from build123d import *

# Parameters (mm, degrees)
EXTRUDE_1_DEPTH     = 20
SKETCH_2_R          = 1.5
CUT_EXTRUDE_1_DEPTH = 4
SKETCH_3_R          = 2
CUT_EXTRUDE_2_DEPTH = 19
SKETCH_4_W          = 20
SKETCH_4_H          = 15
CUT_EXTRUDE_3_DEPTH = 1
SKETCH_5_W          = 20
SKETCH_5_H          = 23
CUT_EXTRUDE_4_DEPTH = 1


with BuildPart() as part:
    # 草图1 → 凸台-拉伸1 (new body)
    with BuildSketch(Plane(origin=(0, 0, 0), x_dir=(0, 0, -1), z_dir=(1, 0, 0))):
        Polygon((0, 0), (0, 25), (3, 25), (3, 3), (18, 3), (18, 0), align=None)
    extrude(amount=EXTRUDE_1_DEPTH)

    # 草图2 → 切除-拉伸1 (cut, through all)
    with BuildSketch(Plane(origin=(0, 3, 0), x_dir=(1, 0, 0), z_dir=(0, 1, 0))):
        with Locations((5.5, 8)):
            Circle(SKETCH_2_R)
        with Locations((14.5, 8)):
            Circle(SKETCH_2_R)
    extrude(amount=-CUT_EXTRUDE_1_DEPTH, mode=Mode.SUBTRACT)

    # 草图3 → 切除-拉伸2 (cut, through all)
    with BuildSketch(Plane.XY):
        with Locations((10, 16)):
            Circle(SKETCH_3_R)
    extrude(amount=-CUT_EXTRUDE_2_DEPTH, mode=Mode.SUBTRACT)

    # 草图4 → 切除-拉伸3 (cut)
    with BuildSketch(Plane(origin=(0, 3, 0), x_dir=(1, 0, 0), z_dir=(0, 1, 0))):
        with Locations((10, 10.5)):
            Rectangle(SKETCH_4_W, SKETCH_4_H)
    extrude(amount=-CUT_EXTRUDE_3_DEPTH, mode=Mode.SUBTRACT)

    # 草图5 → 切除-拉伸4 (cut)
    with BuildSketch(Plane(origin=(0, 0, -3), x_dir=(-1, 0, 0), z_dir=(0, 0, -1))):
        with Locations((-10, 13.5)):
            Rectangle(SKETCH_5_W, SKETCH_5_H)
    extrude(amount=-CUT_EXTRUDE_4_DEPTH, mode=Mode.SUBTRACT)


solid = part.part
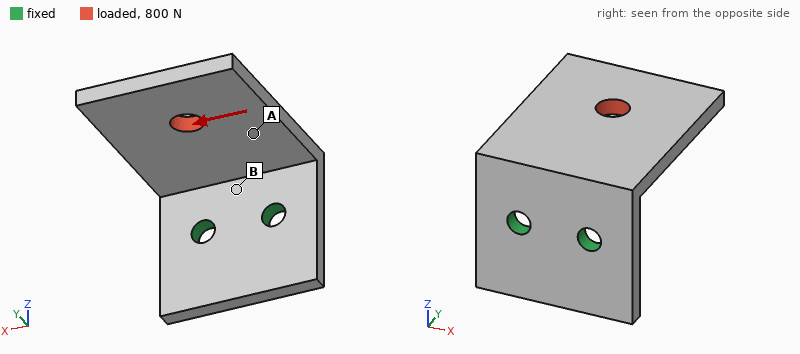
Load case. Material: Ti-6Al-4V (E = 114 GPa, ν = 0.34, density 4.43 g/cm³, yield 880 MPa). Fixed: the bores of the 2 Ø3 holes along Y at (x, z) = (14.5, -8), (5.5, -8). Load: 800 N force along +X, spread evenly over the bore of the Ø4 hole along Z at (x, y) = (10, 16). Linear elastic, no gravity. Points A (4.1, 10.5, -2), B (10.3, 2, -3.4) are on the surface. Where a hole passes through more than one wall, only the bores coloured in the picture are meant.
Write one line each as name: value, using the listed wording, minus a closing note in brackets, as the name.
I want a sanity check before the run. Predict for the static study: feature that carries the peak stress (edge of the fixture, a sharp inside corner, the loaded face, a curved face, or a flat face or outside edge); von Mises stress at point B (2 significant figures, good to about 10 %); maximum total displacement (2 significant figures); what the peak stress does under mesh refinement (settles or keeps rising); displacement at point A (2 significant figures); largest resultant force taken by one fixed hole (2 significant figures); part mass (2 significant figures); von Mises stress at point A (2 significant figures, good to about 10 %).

feature that carries the peak stress: edge of the fixture
von Mises stress at point B: 340 MPa
maximum total displacement: 0.31 mm
what the peak stress does under mesh refinement: keeps rising
displacement at point A: 0.14 mm
largest resultant force taken by one fixed hole: 1.2 kN
part mass: 7.0 g
von Mises stress at point A: 89 MPa
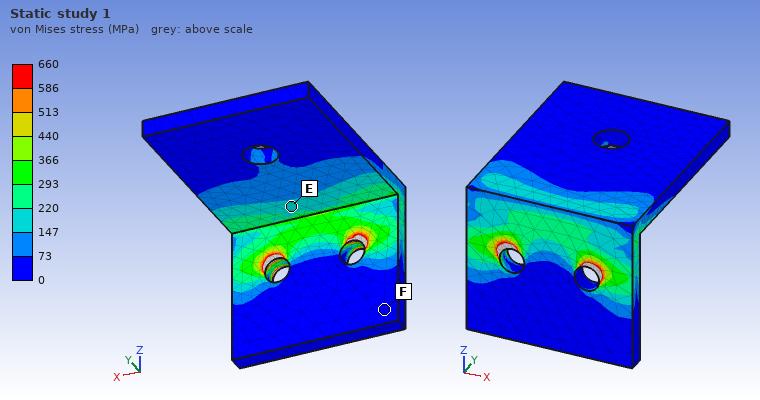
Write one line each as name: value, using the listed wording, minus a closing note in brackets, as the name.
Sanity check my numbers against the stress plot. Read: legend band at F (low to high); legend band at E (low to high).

legend band at F: 0 to 73 MPa
legend band at E: 147 to 220 MPa
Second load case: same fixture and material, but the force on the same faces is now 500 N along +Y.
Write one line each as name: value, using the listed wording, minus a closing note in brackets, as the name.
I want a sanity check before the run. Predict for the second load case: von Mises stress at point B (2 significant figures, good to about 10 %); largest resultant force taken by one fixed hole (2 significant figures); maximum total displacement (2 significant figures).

von Mises stress at point B: 82 MPa
largest resultant force taken by one fixed hole: 250 N
maximum total displacement: 0.16 mm
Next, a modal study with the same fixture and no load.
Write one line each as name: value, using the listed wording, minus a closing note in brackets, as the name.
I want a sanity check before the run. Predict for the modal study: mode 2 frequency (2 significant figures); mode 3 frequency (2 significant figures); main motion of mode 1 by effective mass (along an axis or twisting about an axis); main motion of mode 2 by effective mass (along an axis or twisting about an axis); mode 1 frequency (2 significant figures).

mode 2 frequency: 5100 Hz
mode 3 frequency: 7600 Hz
main motion of mode 1 by effective mass: along Z
main motion of mode 2 by effective mass: along X
mode 1 frequency: 2100 Hz
